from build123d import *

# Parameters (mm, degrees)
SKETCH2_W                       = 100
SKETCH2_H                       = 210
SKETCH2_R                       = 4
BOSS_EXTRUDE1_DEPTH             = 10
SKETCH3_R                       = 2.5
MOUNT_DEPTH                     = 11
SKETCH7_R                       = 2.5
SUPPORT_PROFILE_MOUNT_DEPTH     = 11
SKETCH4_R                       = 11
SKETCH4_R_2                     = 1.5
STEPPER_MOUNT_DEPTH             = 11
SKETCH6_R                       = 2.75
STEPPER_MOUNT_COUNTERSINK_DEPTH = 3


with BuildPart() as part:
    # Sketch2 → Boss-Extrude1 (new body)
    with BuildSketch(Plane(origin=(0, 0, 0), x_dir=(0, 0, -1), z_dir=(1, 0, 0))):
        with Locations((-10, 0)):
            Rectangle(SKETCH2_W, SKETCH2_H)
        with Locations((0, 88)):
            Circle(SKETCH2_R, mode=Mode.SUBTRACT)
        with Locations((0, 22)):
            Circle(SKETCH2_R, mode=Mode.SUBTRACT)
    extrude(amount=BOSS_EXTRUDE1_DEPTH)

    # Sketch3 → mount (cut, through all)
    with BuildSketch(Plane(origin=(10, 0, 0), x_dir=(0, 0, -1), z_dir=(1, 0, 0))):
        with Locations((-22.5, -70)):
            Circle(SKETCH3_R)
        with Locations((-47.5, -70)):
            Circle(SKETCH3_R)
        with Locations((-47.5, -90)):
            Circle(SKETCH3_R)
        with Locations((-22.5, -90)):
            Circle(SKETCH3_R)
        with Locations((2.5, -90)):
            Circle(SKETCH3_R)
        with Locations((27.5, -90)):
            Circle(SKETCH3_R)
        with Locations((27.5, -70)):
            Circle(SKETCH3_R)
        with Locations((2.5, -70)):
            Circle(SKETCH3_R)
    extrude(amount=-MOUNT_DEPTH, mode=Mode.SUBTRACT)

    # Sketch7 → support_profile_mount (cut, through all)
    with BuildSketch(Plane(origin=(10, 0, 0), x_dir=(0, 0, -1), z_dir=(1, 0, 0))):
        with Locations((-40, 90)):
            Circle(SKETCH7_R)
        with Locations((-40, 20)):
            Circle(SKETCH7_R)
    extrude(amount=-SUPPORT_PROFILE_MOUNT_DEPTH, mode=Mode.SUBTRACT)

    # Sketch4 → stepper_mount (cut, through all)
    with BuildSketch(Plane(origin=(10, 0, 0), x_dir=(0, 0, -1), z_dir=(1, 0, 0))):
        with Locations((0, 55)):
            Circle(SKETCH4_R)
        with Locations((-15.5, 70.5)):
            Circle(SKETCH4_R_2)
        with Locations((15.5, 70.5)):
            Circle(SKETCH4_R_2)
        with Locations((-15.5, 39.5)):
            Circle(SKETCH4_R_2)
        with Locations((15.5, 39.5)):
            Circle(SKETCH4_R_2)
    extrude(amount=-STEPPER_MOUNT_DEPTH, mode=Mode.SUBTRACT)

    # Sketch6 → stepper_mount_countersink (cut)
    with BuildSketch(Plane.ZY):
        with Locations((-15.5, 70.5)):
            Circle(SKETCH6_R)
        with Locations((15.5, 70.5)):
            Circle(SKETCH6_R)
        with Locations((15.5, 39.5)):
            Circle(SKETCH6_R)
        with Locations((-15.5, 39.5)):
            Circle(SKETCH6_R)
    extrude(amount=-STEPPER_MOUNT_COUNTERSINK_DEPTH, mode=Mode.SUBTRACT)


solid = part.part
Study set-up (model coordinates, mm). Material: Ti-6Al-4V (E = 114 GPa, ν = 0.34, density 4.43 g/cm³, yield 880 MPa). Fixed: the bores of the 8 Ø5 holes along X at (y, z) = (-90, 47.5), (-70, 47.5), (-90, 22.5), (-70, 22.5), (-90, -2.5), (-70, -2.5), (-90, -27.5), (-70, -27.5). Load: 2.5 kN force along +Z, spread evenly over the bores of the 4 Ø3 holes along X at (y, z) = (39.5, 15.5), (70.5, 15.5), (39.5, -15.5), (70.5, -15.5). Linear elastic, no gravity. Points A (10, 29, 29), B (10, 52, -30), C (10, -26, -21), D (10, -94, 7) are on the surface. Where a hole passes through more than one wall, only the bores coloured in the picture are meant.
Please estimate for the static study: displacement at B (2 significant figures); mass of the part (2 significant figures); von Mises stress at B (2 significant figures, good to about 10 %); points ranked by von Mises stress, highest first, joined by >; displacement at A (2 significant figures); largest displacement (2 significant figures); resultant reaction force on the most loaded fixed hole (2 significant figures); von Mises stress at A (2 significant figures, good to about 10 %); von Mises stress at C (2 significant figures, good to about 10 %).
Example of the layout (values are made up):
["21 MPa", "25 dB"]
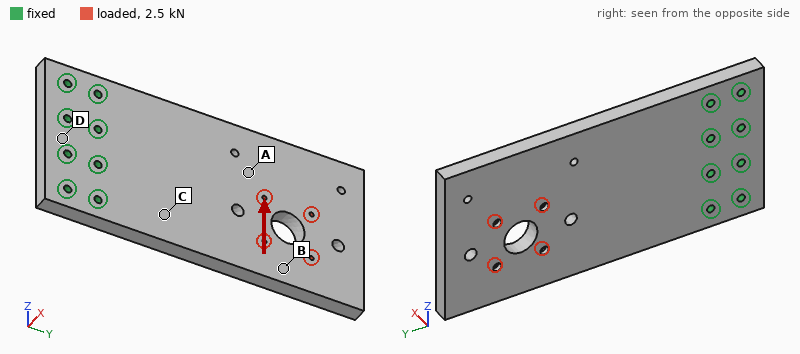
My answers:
["32 µm", "900 g", "4.1 MPa", "C > A > B > D", "22 µm", "46 µm", "3.0 kN", "6.6 MPa", "9.2 MPa"]
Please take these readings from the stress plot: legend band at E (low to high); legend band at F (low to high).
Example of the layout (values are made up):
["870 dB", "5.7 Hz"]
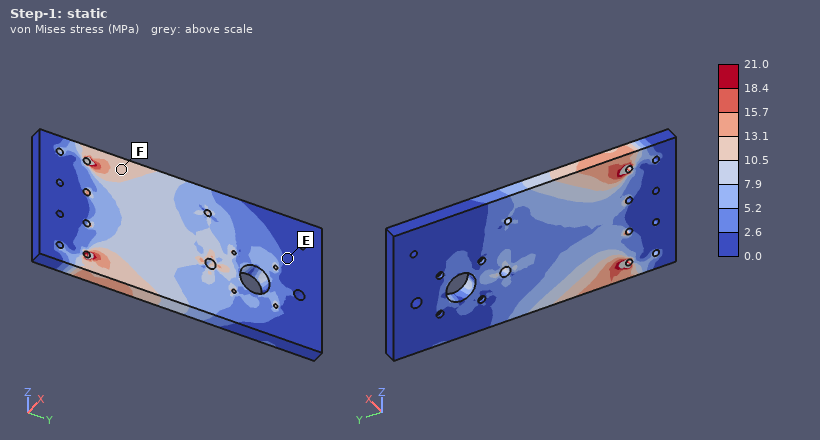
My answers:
["0.0 to 2.6 MPa", "10.5 to 13.1 MPa"]
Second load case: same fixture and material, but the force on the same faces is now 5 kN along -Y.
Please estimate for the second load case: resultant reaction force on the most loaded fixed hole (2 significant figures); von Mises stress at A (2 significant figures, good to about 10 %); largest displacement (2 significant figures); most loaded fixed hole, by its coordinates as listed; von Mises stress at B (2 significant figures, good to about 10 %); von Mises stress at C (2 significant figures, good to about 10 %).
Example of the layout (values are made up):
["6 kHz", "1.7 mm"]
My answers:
["1.6 kN", "8.9 MPa", "0.11 mm", "(-70, -27.5)", "7.4 MPa", "11 MPa"]
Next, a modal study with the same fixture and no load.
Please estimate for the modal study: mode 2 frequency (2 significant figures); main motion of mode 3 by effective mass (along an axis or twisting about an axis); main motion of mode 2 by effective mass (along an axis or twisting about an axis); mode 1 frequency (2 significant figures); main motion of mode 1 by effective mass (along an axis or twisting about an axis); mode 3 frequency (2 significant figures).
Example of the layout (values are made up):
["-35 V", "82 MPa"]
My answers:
["980 Hz", "along X", "twisting about Y", "280 Hz", "along X", "1600 Hz"]
